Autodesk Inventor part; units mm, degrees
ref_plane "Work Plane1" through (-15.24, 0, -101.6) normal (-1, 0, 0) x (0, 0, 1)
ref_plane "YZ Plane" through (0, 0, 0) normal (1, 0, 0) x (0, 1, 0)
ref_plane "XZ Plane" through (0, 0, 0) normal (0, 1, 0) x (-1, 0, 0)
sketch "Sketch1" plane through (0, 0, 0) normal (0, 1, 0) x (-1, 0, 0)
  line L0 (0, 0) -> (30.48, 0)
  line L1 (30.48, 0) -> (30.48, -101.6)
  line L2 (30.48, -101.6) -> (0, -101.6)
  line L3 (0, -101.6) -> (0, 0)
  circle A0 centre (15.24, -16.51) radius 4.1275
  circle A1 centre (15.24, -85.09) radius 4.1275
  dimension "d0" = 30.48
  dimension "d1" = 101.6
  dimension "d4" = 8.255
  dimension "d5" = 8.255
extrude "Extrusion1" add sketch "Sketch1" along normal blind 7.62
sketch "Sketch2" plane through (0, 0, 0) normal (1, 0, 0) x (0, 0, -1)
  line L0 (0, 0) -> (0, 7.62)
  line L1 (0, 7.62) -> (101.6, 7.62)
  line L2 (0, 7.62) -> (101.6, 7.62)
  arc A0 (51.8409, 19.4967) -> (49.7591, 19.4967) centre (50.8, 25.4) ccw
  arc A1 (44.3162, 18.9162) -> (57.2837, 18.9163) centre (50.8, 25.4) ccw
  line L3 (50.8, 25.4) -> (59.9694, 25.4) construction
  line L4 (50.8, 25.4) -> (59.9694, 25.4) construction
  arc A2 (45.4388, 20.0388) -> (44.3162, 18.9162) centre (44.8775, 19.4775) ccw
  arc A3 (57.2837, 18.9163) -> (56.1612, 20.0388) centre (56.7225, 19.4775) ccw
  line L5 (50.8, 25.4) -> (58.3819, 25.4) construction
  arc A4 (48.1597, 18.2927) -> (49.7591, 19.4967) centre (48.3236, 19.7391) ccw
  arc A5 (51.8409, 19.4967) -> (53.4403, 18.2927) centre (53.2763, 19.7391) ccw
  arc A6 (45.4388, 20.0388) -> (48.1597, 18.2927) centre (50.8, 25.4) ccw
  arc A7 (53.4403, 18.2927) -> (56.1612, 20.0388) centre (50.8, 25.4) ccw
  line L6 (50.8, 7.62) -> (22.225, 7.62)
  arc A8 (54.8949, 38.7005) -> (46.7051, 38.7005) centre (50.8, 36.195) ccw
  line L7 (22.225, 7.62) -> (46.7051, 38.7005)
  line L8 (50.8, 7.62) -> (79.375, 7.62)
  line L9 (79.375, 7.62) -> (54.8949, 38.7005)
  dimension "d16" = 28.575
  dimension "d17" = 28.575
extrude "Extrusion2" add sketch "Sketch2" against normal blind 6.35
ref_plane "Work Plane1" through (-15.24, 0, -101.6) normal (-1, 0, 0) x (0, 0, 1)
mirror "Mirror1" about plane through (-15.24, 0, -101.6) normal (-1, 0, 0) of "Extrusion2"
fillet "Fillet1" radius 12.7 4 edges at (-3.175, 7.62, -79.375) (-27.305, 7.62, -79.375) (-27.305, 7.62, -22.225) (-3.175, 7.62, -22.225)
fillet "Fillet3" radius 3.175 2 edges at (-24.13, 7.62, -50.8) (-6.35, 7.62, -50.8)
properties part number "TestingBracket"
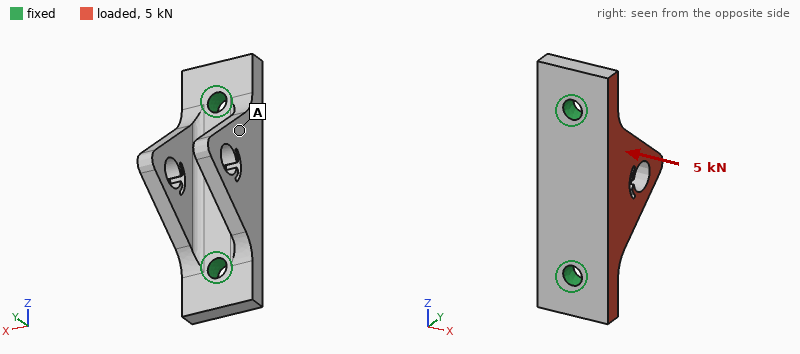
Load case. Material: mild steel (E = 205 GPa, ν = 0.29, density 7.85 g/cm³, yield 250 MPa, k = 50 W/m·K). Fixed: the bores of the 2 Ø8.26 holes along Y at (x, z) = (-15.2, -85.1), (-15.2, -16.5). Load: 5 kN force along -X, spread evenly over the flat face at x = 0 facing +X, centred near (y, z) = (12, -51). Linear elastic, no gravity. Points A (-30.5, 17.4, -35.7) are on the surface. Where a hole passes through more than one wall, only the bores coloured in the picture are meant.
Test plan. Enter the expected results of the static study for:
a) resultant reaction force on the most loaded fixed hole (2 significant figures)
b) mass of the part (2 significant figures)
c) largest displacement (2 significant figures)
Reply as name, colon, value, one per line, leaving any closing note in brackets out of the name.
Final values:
resultant reaction force on the most loaded fixed hole: 2.5 kN
mass of the part: 270 g
largest displacement: 0.11 mm
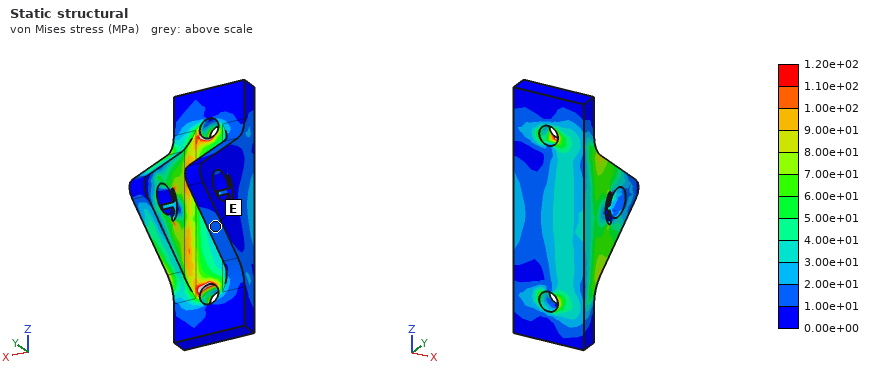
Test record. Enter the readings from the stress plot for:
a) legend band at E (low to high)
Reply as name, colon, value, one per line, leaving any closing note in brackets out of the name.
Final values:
legend band at E: 1.00e+01 to 2.00e+01 MPa
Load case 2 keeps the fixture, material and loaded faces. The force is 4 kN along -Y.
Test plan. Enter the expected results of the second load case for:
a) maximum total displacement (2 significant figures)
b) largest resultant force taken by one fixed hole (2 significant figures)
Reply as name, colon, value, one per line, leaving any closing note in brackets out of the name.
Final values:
maximum total displacement: 58 µm
largest resultant force taken by one fixed hole: 2.1 kN
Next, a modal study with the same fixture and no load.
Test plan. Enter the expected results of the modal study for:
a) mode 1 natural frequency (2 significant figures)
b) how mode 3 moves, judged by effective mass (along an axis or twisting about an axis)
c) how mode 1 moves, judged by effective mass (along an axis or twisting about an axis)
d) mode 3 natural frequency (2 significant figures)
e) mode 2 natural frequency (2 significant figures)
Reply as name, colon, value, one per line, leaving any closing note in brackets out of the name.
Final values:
mode 1 natural frequency: 4600 Hz
how mode 3 moves, judged by effective mass: along Y
how mode 1 moves, judged by effective mass: along X
mode 3 natural frequency: 9500 Hz
mode 2 natural frequency: 5800 Hz
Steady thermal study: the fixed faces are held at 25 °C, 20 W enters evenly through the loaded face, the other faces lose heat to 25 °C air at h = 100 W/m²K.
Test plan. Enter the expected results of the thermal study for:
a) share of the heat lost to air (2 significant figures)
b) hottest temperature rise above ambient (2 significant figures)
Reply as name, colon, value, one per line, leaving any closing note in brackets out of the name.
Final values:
share of the heat lost to air: 32 %
hottest temperature rise above ambient: 21 K
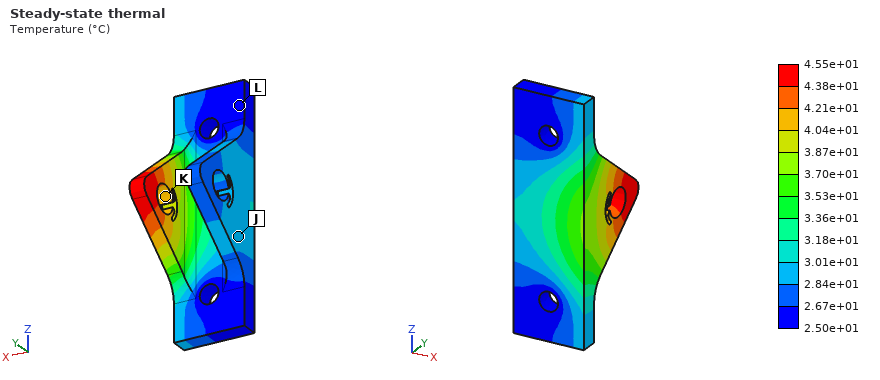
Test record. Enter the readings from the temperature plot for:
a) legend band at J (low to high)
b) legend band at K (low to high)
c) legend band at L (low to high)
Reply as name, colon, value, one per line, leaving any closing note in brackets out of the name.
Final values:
legend band at J: 2.84e+01 to 3.01e+01 °C
legend band at K: 4.04e+01 to 4.21e+01 °C
legend band at L: 2.50e+01 to 2.67e+01 °C
